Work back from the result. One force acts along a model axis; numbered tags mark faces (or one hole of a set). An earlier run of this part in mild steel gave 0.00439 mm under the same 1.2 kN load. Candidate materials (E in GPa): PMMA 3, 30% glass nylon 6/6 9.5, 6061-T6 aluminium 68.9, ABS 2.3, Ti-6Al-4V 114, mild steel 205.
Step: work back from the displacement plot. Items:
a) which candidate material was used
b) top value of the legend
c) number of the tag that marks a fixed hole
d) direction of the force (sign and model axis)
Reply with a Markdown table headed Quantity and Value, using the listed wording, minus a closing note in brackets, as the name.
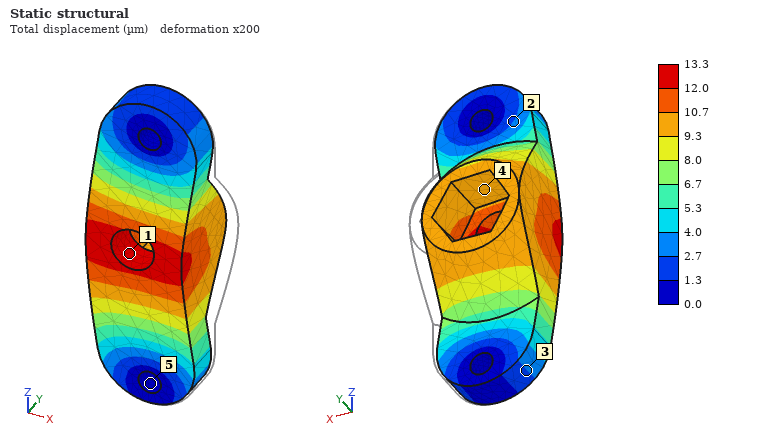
| Quantity | Value |
|---|---|
| which candidate material was used | 6061-T6 aluminium |
| top value of the legend | 13.3 µm |
| number of the tag that marks a fixed hole | 5 |
| direction of the force | -X |
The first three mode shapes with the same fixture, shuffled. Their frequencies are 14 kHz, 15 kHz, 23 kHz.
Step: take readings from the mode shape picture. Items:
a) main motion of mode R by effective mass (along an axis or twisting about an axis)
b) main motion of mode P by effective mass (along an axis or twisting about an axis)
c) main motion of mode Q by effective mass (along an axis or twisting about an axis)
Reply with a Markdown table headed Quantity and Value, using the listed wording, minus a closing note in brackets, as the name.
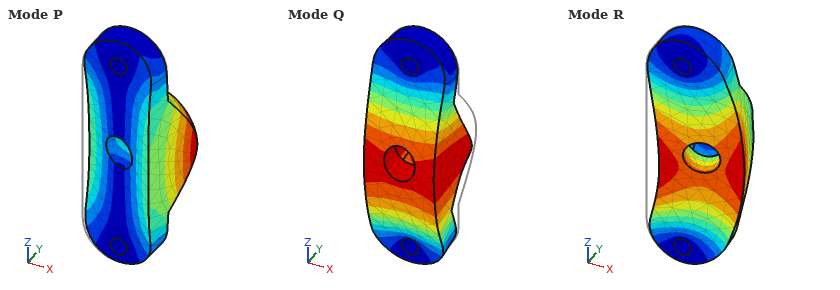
| Quantity | Value |
|---|---|
| main motion of mode R by effective mass | along X |
| main motion of mode P by effective mass | along X |
| main motion of mode Q by effective mass | along Y |
